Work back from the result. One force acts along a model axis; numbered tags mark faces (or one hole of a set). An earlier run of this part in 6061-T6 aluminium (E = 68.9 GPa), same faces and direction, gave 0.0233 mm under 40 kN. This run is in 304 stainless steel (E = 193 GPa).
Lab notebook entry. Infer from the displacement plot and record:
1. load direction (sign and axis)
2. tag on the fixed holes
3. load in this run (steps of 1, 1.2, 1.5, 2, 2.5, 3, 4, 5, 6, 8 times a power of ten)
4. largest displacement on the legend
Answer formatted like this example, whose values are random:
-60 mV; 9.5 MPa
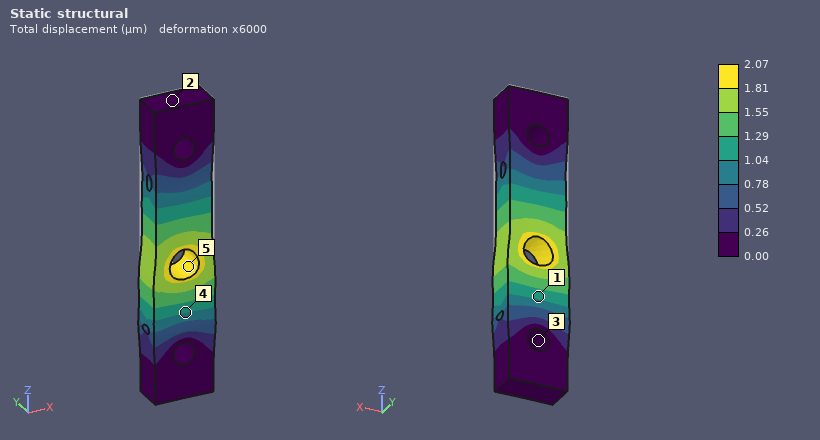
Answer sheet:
-Z; 3; 10 kN; 2.07 µm
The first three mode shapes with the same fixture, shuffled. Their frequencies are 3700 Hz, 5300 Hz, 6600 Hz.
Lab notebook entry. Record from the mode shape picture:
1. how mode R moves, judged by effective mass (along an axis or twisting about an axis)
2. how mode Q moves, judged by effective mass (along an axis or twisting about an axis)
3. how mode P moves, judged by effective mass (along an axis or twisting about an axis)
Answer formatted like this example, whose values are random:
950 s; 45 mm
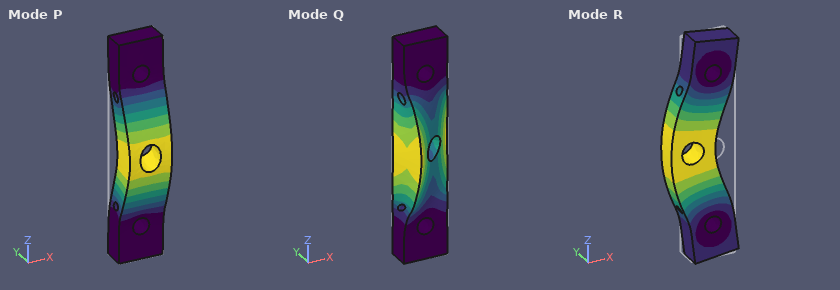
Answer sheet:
along X; twisting about Z; along Y
